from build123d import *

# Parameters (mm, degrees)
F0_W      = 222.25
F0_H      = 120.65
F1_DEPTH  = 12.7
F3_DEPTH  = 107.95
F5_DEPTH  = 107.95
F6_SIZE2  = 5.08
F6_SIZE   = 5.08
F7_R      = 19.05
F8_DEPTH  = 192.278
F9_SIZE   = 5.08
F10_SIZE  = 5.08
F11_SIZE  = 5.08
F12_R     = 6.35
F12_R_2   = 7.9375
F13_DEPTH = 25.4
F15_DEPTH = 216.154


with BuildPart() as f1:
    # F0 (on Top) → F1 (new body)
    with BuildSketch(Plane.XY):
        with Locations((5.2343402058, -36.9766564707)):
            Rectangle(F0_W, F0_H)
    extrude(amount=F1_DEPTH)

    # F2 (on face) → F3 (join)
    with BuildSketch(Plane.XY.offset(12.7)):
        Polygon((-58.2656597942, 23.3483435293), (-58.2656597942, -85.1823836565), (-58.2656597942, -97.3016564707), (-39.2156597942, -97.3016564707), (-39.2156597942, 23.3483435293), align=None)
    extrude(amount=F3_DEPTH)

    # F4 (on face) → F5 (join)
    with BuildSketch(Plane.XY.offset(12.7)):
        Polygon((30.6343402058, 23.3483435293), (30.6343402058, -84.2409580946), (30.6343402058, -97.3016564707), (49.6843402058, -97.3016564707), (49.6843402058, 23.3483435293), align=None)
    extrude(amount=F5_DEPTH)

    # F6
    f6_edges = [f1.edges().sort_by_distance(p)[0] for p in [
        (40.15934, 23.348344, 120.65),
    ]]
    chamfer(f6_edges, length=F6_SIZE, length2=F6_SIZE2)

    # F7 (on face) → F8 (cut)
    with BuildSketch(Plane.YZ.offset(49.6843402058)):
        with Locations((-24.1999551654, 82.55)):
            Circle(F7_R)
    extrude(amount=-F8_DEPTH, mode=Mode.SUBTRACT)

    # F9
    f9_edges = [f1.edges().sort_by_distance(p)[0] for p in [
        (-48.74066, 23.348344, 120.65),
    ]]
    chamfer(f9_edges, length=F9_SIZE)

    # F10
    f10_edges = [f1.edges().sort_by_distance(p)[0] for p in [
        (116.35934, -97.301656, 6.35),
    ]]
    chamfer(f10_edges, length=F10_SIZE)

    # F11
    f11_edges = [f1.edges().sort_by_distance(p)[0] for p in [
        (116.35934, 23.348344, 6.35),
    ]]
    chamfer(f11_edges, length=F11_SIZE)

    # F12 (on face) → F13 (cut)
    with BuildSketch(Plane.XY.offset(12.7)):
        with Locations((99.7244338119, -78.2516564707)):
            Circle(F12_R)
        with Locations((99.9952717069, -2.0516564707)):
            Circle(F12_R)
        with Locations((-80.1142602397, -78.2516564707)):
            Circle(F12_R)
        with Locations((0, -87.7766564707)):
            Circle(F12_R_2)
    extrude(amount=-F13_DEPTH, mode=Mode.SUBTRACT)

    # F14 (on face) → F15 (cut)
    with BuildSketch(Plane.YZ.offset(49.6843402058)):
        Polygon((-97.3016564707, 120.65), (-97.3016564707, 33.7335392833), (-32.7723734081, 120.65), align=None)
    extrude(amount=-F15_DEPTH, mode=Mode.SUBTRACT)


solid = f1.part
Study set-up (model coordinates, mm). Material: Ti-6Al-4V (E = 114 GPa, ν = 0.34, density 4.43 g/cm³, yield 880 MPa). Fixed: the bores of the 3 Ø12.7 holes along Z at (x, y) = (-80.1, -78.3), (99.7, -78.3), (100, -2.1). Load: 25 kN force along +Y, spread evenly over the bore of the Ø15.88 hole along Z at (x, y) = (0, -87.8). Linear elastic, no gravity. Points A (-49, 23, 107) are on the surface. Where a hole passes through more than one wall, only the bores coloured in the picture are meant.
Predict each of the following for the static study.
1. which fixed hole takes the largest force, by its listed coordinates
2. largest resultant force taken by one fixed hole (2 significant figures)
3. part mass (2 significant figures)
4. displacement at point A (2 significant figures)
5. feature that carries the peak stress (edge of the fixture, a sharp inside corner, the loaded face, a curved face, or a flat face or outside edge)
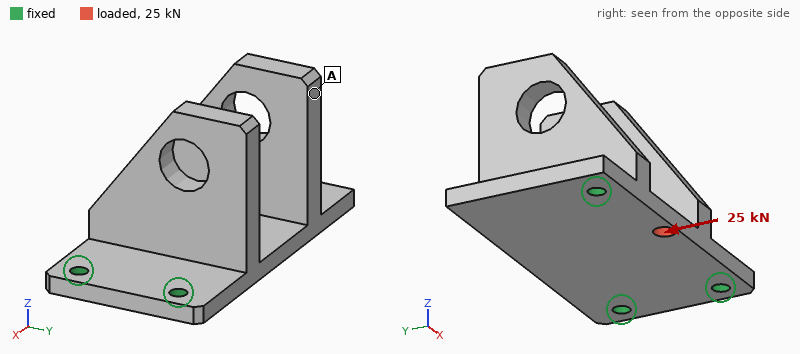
(-80.1, -78.3)
12 kN
3.0 kg
21 µm
a flat face or outside edge
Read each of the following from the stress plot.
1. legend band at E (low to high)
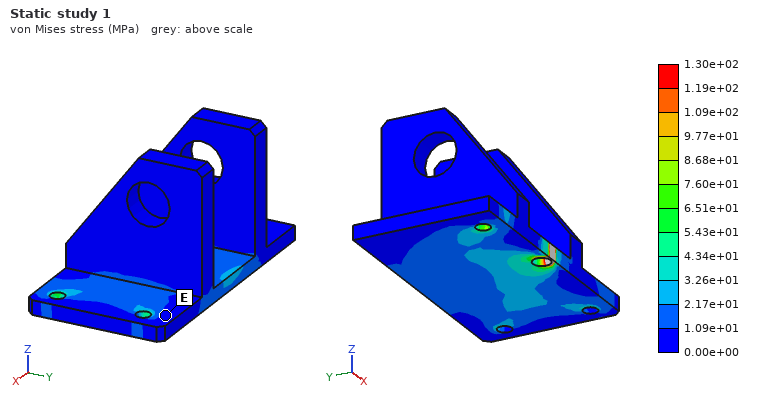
0.00e+00 to 1.09e+01 MPa
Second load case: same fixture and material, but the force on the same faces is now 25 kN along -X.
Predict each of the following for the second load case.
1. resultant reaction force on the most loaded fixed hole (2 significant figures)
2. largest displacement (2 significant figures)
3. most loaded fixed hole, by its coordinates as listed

12 kN
28 µm
(-80.1, -78.3)
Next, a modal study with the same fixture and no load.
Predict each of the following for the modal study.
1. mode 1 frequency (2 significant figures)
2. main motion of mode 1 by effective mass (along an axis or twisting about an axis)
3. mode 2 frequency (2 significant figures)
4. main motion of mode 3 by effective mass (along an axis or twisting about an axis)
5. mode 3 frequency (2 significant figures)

640 Hz
along Z
820 Hz
along X
1300 Hz
